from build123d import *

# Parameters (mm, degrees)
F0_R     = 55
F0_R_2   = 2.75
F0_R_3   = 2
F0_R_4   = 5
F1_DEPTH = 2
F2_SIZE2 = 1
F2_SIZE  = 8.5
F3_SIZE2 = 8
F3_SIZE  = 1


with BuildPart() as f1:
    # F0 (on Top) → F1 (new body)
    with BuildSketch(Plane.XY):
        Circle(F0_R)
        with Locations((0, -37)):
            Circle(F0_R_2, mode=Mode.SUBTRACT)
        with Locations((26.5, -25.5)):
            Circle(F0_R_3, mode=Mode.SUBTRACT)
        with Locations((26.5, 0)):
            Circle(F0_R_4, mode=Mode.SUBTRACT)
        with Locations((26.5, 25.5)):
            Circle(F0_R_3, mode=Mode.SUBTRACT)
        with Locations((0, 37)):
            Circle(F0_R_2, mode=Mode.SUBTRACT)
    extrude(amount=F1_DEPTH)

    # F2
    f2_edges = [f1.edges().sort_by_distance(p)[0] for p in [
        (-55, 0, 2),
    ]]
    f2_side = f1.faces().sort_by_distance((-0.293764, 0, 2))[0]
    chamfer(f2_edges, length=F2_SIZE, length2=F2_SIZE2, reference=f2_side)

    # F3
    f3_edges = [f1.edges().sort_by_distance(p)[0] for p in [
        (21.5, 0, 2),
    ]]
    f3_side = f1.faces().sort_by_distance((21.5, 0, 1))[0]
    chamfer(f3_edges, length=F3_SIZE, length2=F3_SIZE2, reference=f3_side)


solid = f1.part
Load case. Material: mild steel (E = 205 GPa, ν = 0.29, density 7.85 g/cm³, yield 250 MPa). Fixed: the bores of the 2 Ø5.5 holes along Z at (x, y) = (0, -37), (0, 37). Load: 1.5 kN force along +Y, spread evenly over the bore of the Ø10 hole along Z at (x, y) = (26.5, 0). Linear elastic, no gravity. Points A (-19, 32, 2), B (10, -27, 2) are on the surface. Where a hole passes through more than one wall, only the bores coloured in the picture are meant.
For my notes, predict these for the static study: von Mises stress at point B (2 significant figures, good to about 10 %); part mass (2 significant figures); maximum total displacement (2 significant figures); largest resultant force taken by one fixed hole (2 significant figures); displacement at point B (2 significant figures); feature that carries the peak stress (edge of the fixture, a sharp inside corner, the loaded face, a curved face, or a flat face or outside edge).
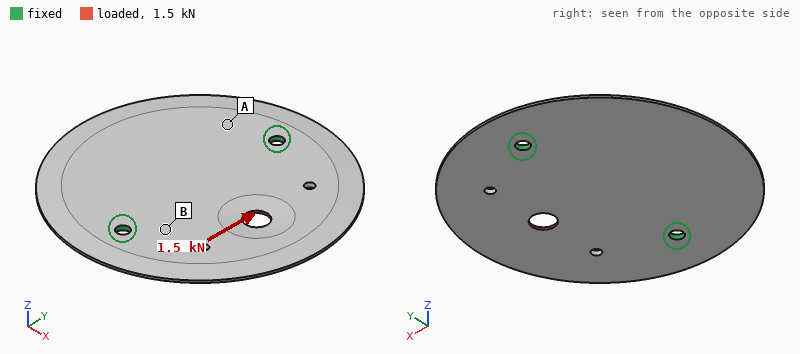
17 MPa
130 g
17 µm
910 N
3.2 µm
the loaded face
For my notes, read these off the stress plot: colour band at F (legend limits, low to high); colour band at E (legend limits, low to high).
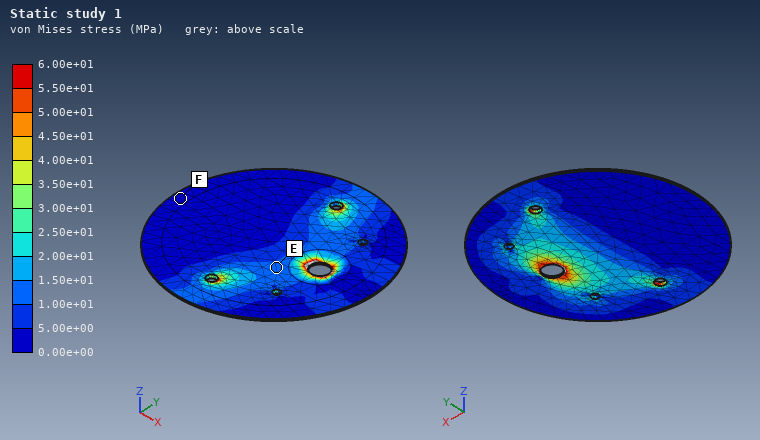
0.00e+00 to 5.00e+00 MPa
1.00e+01 to 1.50e+01 MPa
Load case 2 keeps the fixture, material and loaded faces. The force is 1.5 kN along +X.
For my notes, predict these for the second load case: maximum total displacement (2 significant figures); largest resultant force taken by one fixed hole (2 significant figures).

88 µm
760 N
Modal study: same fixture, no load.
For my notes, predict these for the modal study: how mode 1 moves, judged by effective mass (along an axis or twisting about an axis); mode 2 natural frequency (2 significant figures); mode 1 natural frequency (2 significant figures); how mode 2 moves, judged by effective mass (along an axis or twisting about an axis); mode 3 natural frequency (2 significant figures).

twisting about Y
720 Hz
570 Hz
along Z
1500 Hz
